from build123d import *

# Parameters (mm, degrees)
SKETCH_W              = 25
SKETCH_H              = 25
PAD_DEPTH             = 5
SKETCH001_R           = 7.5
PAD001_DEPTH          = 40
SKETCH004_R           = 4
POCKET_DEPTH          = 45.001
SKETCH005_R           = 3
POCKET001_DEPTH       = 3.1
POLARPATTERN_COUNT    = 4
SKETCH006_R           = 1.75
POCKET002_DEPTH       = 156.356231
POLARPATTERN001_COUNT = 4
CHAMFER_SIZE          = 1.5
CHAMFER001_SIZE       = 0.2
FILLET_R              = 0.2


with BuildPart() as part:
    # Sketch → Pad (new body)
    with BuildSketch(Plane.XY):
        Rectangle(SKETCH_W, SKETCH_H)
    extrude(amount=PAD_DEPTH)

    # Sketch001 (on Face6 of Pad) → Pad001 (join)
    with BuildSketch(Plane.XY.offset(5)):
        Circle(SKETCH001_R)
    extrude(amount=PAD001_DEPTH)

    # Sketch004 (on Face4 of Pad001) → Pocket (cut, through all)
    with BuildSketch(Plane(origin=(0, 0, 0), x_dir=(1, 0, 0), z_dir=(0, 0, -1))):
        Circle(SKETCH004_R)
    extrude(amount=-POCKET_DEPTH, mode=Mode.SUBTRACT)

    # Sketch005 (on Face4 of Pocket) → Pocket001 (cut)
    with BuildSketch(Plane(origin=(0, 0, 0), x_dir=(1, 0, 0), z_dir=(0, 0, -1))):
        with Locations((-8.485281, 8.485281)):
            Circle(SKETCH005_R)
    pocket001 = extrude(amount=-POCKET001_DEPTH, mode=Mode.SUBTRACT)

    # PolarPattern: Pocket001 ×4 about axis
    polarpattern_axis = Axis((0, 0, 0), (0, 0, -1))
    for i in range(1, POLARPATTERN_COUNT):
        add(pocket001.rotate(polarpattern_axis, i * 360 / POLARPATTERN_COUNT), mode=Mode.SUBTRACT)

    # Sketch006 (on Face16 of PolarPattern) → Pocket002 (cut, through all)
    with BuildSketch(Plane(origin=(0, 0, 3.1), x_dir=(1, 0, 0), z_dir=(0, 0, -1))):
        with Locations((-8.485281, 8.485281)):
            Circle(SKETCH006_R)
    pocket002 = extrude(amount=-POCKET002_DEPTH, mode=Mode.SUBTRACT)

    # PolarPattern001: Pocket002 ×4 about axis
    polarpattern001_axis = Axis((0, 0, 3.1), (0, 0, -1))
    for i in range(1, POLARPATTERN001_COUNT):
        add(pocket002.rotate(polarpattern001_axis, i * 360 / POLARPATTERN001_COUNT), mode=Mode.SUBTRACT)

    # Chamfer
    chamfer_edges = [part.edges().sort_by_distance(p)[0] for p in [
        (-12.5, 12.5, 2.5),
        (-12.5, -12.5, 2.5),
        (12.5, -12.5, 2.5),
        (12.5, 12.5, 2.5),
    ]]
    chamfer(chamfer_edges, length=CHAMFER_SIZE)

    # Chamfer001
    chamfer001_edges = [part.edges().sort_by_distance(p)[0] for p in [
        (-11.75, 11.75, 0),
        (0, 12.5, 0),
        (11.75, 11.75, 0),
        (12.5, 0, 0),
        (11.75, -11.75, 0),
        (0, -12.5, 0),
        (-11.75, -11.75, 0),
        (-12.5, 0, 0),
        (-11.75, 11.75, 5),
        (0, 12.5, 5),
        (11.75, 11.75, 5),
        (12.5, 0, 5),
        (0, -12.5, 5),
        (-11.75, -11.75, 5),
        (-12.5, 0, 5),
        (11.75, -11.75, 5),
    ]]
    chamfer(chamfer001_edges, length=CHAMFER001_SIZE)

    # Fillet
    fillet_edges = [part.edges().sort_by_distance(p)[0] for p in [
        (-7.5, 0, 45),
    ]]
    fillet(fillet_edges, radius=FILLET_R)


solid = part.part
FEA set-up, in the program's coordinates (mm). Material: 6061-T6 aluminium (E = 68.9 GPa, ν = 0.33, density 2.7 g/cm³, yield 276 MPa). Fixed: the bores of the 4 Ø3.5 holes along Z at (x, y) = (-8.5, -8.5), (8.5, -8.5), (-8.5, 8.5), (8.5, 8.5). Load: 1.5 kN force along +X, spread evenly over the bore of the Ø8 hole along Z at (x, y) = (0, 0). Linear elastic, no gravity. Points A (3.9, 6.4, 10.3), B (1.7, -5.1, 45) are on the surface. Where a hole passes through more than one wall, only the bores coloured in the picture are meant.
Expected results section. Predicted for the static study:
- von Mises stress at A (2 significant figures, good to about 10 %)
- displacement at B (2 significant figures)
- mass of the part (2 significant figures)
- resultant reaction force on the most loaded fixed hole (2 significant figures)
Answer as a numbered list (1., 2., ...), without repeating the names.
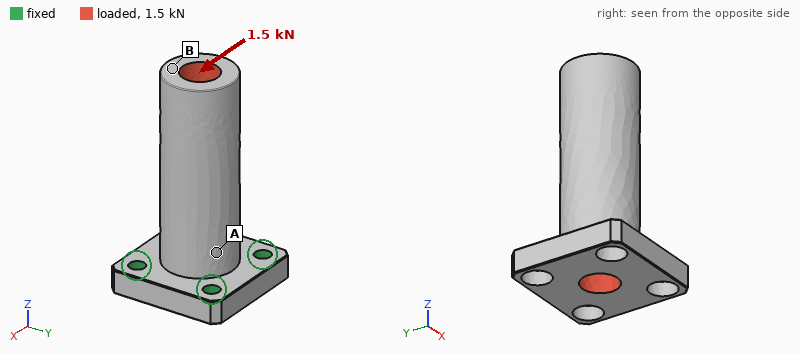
1. 37 MPa
2. 0.16 mm
3. 20 g
4. 940 N
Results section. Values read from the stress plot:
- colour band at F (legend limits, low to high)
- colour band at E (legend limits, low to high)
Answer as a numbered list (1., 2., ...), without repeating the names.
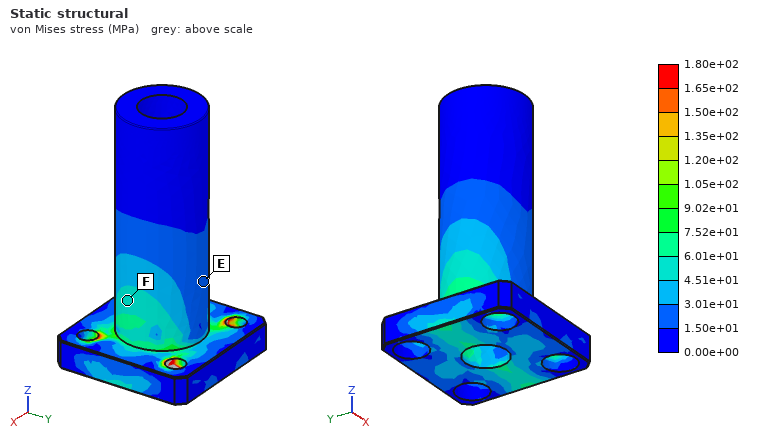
1. 4.51e+01 to 6.01e+01 MPa
2. 1.50e+01 to 3.01e+01 MPa
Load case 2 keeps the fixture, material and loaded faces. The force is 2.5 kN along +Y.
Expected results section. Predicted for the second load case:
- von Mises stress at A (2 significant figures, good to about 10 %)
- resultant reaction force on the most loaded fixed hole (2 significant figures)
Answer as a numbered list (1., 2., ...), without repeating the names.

1. 92 MPa
2. 1.6 kN
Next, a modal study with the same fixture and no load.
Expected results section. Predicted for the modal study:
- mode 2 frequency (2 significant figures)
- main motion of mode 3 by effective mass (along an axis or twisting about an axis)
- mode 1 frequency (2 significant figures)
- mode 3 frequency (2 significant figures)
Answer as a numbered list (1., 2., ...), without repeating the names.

1. 4800 Hz
2. twisting about Z
3. 4800 Hz
4. 18 kHz
